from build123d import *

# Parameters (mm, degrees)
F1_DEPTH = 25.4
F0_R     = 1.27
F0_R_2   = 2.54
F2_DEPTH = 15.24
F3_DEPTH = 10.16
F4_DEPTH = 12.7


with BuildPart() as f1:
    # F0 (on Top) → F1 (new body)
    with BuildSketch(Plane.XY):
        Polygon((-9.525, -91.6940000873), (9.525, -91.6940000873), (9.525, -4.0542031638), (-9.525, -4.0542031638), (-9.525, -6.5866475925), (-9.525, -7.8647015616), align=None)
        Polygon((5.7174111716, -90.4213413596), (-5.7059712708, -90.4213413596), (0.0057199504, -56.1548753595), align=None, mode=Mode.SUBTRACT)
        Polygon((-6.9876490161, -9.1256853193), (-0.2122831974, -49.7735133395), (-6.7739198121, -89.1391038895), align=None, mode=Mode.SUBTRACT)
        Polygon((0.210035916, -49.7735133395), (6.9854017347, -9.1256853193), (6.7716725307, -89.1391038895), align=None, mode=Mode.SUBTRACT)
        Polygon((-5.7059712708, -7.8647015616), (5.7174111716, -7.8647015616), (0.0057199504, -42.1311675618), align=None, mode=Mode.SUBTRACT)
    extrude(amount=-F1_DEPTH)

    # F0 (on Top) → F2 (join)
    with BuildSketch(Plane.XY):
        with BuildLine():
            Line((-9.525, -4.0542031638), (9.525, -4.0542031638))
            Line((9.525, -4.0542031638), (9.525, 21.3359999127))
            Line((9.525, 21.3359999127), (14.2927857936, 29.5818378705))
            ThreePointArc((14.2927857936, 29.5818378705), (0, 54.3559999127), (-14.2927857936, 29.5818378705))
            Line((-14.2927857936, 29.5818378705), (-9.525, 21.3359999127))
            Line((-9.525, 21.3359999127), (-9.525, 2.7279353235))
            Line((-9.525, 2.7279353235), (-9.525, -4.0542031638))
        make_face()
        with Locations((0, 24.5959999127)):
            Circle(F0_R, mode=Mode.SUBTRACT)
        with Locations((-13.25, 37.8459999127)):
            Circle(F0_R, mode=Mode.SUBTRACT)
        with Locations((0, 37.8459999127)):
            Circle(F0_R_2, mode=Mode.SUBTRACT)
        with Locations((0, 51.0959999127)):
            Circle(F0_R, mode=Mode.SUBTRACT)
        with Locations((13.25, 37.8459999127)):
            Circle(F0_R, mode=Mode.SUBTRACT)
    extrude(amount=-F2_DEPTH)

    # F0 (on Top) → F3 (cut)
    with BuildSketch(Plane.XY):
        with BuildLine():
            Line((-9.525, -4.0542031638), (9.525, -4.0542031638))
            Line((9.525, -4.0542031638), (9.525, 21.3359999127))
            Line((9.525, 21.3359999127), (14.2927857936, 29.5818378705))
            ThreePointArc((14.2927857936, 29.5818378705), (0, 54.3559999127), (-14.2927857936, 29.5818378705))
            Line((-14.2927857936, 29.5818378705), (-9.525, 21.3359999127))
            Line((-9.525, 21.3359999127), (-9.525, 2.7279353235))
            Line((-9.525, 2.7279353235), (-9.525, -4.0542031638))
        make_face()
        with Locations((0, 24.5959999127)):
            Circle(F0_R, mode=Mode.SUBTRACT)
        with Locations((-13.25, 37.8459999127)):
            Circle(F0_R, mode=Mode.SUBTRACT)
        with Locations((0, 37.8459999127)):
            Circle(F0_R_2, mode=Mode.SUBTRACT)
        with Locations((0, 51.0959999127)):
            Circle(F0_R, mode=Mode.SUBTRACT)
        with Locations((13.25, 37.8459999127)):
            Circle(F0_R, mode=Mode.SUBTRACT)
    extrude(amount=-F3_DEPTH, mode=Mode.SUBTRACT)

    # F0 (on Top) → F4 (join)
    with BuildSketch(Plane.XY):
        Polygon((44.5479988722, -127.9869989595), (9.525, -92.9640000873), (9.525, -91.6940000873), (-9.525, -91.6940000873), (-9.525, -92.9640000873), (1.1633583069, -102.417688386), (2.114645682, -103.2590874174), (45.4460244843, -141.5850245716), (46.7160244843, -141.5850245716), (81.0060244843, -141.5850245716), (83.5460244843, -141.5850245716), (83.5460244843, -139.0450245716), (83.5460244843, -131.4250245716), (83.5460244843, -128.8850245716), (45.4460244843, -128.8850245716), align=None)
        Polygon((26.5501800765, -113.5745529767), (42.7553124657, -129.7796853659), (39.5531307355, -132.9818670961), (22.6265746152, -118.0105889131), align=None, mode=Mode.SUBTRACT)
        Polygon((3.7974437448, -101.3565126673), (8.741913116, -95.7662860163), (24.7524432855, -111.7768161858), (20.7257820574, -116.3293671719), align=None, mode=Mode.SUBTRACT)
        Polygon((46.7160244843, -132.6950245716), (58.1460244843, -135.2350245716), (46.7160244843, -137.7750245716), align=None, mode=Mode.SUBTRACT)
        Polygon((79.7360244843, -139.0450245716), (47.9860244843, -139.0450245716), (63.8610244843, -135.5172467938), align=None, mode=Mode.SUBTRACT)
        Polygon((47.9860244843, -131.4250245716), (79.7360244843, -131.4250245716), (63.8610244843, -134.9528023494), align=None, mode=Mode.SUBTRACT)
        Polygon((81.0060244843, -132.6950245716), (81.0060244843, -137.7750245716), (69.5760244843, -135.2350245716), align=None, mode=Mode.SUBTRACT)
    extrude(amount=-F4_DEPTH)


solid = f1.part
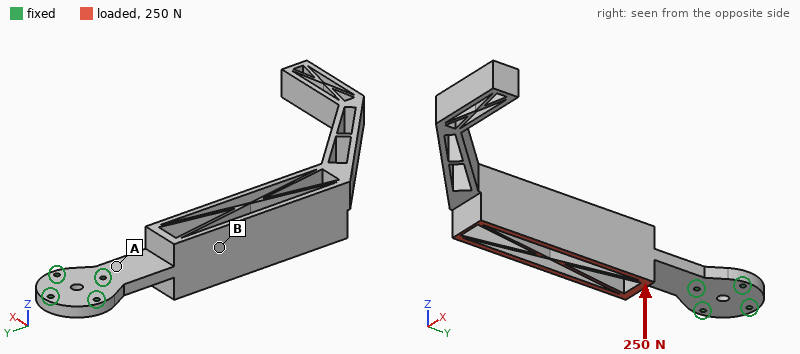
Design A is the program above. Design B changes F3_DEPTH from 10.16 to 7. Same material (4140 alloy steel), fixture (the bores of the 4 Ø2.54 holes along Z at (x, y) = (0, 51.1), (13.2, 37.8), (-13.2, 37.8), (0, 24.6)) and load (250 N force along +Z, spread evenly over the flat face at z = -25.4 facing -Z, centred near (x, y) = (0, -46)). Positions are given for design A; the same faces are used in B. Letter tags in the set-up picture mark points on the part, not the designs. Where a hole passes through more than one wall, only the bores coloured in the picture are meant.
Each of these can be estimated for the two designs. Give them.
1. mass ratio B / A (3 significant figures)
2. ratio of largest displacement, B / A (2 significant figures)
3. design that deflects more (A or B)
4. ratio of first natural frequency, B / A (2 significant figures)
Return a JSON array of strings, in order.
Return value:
["1.12", "0.26", "A", "1.8"]
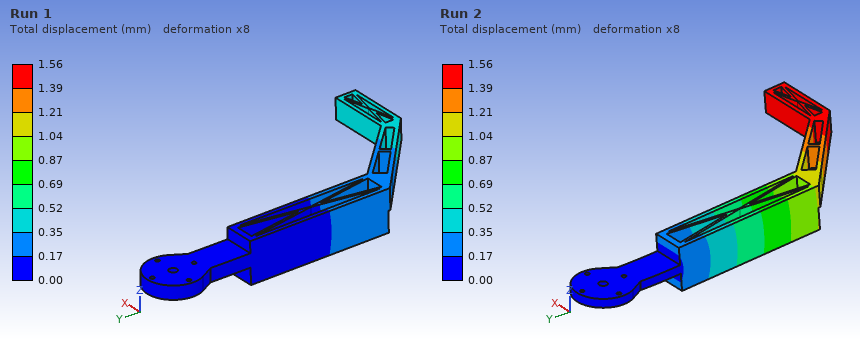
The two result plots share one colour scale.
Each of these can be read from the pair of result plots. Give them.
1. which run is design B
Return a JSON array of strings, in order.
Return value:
["Run 1"]
